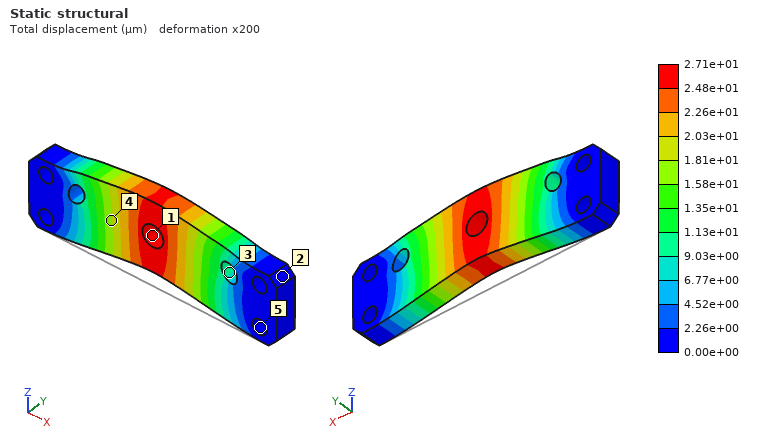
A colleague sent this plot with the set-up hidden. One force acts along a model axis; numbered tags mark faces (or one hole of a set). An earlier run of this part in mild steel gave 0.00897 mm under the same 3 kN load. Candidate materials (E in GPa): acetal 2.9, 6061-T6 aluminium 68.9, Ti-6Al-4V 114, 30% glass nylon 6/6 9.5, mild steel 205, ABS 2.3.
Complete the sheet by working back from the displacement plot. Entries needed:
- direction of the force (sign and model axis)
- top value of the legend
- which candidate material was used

+Z
2.71e+01 µm
6061-T6 aluminium
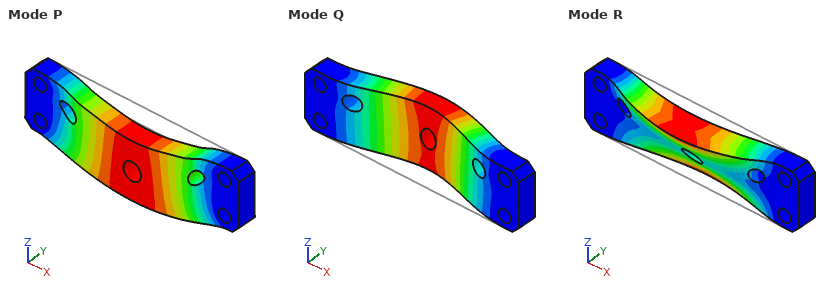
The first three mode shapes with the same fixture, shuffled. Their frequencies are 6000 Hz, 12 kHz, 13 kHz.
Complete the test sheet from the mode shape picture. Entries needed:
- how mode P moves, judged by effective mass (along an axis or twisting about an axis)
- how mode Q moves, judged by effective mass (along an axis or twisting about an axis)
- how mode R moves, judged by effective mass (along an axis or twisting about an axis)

along Z
along Y
twisting about X
